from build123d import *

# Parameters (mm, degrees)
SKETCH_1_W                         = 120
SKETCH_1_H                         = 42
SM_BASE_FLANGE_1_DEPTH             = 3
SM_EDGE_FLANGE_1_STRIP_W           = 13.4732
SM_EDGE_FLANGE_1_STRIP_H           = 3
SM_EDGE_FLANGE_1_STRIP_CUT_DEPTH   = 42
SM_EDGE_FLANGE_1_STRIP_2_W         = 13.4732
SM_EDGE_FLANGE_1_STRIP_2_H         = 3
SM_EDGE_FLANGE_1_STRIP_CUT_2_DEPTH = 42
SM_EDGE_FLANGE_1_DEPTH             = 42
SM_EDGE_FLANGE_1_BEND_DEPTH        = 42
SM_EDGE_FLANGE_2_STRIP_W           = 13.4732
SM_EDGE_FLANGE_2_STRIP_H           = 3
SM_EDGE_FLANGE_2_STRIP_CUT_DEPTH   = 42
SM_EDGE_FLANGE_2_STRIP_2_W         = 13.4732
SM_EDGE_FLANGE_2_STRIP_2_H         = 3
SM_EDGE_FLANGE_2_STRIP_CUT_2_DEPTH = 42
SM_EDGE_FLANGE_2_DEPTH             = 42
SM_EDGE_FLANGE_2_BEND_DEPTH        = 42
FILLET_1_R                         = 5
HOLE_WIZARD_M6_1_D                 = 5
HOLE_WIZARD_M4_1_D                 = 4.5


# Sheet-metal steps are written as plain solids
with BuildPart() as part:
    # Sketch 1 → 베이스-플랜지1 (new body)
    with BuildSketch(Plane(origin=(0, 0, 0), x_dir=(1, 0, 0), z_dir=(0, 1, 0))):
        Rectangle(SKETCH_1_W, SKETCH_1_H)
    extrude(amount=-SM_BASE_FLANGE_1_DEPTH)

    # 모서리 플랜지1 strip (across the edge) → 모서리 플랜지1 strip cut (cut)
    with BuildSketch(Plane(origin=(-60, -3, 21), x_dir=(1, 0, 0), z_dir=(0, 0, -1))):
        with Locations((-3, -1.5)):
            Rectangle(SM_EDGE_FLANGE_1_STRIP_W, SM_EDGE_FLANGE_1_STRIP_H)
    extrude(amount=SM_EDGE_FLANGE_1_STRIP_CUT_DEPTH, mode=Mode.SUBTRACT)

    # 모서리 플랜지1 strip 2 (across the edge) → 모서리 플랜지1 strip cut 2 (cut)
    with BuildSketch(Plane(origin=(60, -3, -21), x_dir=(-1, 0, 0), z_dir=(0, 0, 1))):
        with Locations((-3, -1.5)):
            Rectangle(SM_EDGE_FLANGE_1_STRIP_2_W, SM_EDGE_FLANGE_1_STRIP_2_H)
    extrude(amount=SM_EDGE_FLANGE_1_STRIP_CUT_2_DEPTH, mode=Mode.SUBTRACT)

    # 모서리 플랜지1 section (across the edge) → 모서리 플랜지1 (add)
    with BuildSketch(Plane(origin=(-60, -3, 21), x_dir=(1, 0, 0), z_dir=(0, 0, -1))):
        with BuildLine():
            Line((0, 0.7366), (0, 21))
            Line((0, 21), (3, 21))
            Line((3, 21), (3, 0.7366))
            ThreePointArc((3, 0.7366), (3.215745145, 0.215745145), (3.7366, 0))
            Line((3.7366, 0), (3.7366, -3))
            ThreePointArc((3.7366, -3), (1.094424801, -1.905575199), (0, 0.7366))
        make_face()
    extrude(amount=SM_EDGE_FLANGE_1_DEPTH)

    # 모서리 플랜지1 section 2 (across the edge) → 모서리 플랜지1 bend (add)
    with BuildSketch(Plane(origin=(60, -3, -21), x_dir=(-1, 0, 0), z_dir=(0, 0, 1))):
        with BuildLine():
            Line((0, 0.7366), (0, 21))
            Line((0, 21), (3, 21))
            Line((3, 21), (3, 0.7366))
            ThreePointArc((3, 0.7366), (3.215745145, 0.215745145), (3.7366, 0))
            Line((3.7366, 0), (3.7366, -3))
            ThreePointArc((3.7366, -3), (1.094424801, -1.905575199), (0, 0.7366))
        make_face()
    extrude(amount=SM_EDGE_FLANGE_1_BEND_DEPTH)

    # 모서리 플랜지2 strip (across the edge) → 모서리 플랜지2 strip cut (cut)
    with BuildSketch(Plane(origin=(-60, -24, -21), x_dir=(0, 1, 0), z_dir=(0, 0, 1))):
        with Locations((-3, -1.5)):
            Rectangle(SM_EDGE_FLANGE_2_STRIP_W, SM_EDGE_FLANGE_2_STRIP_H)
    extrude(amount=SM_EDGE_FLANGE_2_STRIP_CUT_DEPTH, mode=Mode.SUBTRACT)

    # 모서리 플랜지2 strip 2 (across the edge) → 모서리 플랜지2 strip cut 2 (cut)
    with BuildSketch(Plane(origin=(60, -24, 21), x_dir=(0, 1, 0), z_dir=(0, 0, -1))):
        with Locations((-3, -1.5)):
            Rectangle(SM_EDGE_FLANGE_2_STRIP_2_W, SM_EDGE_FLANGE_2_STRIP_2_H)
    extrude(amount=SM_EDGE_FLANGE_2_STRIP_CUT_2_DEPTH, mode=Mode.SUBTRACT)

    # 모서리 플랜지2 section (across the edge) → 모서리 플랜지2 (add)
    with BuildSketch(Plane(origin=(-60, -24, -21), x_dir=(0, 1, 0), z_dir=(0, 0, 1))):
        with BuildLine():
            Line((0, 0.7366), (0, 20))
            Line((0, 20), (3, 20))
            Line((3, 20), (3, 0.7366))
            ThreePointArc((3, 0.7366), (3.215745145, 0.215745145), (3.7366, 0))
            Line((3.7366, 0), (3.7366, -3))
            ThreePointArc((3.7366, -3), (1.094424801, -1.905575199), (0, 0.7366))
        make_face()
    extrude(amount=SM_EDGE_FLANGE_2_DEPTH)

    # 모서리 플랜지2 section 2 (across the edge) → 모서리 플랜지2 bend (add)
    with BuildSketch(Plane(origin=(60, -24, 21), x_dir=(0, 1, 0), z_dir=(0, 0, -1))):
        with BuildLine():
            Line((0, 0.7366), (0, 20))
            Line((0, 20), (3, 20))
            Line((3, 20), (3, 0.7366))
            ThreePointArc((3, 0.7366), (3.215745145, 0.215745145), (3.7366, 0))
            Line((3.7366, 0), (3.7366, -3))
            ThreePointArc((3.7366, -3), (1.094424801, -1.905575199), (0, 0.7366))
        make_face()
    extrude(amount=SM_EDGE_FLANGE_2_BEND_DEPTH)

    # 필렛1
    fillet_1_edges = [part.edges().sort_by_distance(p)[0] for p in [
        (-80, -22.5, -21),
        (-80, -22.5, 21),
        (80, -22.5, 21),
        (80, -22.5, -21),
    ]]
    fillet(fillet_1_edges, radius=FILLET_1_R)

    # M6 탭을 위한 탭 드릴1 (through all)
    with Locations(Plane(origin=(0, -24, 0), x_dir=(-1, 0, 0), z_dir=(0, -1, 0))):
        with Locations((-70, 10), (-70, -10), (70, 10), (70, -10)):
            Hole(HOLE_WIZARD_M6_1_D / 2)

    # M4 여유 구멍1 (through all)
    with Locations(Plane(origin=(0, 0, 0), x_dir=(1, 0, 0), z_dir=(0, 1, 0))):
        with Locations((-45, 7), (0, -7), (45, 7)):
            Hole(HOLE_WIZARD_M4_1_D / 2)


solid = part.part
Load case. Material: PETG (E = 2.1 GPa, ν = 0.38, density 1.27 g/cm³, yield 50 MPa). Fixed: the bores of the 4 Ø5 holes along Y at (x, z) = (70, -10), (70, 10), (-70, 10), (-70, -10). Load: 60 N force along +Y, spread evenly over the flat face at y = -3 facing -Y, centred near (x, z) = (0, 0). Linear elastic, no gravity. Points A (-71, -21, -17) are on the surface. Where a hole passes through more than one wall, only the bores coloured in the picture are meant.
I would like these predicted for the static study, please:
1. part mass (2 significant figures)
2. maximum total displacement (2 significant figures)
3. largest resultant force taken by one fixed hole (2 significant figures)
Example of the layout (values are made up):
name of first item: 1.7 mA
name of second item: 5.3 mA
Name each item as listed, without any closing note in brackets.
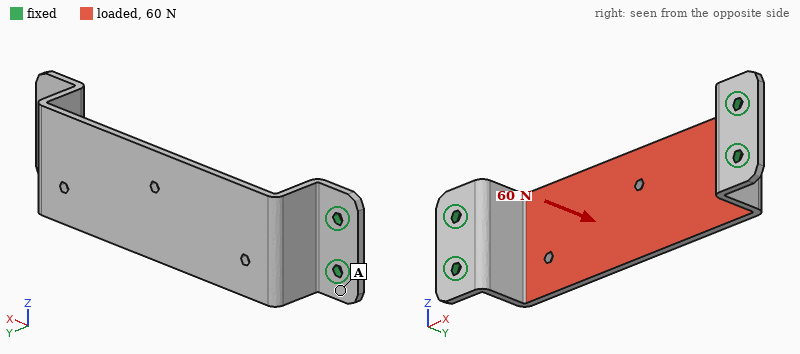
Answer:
part mass: 31 g
maximum total displacement: 1.7 mm
largest resultant force taken by one fixed hole: 24 N
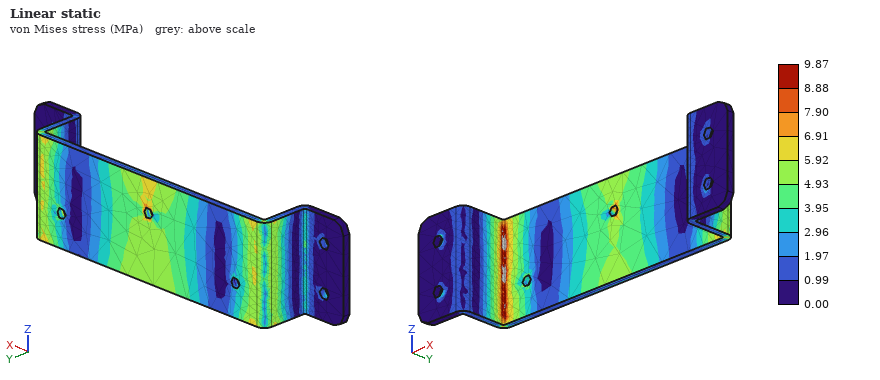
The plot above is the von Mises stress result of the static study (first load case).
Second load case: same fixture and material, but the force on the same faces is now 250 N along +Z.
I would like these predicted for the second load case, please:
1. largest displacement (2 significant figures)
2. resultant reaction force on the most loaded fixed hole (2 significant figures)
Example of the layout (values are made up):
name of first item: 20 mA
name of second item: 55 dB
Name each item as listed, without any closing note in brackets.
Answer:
largest displacement: 0.57 mm
resultant reaction force on the most loaded fixed hole: 140 N
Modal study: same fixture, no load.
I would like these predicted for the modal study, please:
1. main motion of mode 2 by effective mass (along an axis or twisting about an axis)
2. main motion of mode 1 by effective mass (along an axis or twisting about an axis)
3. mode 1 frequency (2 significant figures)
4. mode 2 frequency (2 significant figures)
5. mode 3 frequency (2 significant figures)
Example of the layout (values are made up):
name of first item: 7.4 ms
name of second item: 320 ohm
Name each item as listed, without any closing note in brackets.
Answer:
main motion of mode 2 by effective mass: along X
main motion of mode 1 by effective mass: along Y
mode 1 frequency: 260 Hz
mode 2 frequency: 340 Hz
mode 3 frequency: 520 Hz
